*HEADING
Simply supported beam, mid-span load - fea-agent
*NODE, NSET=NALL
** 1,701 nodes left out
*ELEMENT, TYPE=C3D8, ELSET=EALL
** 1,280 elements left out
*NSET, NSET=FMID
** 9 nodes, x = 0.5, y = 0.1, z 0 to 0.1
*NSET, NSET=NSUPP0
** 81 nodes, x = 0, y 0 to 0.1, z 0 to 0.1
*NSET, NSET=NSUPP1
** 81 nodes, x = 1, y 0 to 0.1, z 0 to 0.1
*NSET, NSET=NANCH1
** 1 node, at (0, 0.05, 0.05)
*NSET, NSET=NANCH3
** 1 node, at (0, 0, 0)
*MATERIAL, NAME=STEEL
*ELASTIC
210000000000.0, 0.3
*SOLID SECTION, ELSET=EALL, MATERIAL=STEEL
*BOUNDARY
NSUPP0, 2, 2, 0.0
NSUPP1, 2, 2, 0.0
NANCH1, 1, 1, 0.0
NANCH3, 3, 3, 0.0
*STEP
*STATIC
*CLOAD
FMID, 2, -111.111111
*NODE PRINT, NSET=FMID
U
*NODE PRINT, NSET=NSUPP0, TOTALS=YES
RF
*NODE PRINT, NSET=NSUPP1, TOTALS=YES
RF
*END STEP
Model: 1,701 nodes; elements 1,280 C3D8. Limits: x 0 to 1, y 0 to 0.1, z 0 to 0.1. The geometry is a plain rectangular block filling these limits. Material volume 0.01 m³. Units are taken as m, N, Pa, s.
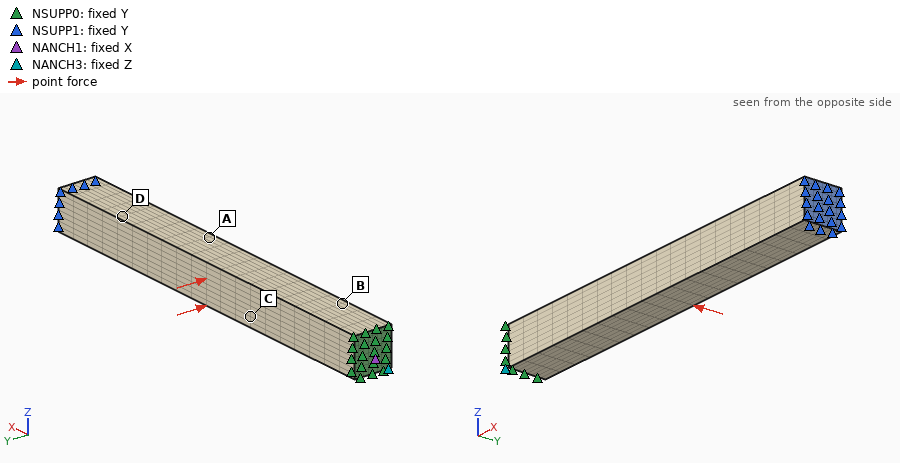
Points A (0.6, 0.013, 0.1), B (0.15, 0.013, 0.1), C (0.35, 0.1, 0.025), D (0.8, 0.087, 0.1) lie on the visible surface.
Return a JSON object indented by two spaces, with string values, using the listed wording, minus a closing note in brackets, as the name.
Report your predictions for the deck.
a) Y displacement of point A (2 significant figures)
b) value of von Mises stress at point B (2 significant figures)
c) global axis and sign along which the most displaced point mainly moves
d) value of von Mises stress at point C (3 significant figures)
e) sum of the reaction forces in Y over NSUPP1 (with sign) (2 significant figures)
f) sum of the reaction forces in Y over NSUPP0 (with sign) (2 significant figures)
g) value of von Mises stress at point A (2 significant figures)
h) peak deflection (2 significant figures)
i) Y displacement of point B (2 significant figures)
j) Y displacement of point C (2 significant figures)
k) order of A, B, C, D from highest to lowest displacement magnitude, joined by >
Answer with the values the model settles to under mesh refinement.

{
  "Y displacement of point A": "-1.2e-05 m",
  "value of von Mises stress at point B": "3.5e+05 Pa",
  "global axis and sign along which the most displaced point mainly moves": "-Y",
  "value of von Mises stress at point C": "1.05e+06 Pa",
  "sum of the reaction forces in Y over NSUPP1 (with sign)": "500 N",
  "sum of the reaction forces in Y over NSUPP0 (with sign)": "500 N",
  "value of von Mises stress at point A": "9.0e+05 Pa",
  "peak deflection": "1.3e-05 m",
  "Y displacement of point B": "-5.3e-06 m",
  "Y displacement of point C": "-1.1e-05 m",
  "order of A, B, C, D from highest to lowest displacement magnitude, joined by >": "A > C > D > B"
}
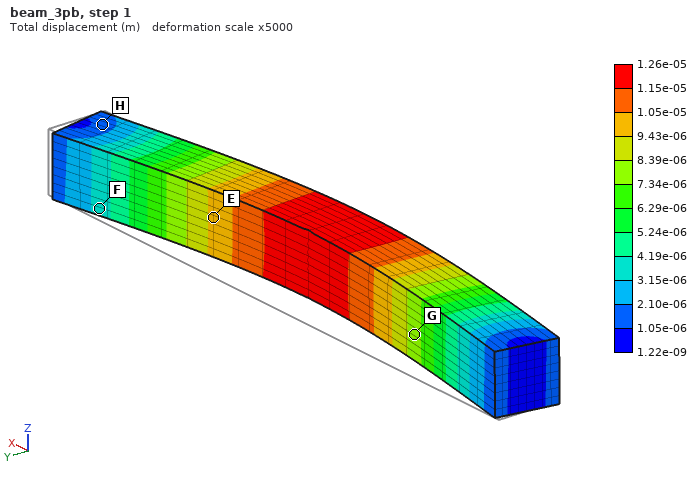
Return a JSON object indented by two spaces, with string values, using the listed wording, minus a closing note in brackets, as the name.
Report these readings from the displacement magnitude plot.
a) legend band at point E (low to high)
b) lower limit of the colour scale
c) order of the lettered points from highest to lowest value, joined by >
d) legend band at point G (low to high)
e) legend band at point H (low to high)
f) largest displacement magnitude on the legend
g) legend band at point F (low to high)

{
  "legend band at point E": "9.43e-06 to 1.05e-05 m",
  "lower limit of the colour scale": "1.22e-09 m",
  "order of the lettered points from highest to lowest value, joined by >": "E > G > F > H",
  "legend band at point G": "7.34e-06 to 8.39e-06 m",
  "legend band at point H": "1.05e-06 to 2.10e-06 m",
  "largest displacement magnitude on the legend": "1.26e-05 m",
  "legend band at point F": "3.15e-06 to 4.19e-06 m"
}
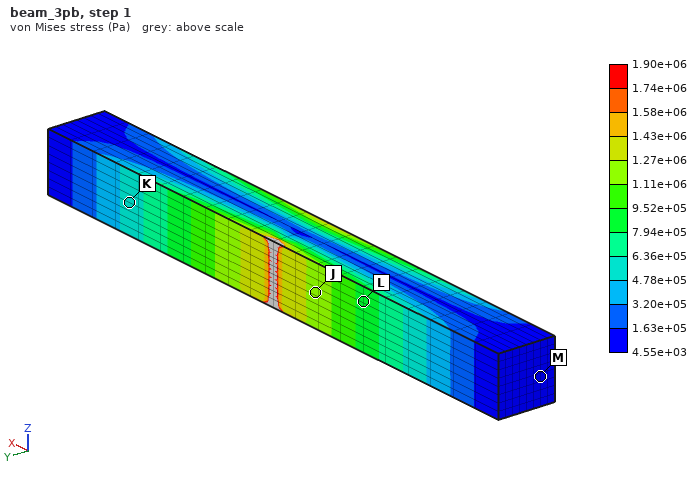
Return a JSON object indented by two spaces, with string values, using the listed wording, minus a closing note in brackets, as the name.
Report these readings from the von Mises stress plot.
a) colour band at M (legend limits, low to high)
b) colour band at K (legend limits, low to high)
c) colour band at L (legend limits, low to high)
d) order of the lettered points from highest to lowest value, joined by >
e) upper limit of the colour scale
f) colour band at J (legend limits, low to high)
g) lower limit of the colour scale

{
  "colour band at M": "4.55e+03 to 1.63e+05 Pa",
  "colour band at K": "4.78e+05 to 6.36e+05 Pa",
  "colour band at L": "7.94e+05 to 9.52e+05 Pa",
  "order of the lettered points from highest to lowest value, joined by >": "J > L > K > M",
  "upper limit of the colour scale": "1.90e+06 Pa",
  "colour band at J": "1.11e+06 to 1.27e+06 Pa",
  "lower limit of the colour scale": "4.55e+03 Pa"
}
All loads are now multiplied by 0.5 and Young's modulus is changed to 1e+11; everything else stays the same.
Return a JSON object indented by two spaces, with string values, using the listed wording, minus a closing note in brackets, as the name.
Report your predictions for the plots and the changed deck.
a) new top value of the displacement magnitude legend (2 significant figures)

{
  "new top value of the displacement magnitude legend": "1.3e-05 m"
}
